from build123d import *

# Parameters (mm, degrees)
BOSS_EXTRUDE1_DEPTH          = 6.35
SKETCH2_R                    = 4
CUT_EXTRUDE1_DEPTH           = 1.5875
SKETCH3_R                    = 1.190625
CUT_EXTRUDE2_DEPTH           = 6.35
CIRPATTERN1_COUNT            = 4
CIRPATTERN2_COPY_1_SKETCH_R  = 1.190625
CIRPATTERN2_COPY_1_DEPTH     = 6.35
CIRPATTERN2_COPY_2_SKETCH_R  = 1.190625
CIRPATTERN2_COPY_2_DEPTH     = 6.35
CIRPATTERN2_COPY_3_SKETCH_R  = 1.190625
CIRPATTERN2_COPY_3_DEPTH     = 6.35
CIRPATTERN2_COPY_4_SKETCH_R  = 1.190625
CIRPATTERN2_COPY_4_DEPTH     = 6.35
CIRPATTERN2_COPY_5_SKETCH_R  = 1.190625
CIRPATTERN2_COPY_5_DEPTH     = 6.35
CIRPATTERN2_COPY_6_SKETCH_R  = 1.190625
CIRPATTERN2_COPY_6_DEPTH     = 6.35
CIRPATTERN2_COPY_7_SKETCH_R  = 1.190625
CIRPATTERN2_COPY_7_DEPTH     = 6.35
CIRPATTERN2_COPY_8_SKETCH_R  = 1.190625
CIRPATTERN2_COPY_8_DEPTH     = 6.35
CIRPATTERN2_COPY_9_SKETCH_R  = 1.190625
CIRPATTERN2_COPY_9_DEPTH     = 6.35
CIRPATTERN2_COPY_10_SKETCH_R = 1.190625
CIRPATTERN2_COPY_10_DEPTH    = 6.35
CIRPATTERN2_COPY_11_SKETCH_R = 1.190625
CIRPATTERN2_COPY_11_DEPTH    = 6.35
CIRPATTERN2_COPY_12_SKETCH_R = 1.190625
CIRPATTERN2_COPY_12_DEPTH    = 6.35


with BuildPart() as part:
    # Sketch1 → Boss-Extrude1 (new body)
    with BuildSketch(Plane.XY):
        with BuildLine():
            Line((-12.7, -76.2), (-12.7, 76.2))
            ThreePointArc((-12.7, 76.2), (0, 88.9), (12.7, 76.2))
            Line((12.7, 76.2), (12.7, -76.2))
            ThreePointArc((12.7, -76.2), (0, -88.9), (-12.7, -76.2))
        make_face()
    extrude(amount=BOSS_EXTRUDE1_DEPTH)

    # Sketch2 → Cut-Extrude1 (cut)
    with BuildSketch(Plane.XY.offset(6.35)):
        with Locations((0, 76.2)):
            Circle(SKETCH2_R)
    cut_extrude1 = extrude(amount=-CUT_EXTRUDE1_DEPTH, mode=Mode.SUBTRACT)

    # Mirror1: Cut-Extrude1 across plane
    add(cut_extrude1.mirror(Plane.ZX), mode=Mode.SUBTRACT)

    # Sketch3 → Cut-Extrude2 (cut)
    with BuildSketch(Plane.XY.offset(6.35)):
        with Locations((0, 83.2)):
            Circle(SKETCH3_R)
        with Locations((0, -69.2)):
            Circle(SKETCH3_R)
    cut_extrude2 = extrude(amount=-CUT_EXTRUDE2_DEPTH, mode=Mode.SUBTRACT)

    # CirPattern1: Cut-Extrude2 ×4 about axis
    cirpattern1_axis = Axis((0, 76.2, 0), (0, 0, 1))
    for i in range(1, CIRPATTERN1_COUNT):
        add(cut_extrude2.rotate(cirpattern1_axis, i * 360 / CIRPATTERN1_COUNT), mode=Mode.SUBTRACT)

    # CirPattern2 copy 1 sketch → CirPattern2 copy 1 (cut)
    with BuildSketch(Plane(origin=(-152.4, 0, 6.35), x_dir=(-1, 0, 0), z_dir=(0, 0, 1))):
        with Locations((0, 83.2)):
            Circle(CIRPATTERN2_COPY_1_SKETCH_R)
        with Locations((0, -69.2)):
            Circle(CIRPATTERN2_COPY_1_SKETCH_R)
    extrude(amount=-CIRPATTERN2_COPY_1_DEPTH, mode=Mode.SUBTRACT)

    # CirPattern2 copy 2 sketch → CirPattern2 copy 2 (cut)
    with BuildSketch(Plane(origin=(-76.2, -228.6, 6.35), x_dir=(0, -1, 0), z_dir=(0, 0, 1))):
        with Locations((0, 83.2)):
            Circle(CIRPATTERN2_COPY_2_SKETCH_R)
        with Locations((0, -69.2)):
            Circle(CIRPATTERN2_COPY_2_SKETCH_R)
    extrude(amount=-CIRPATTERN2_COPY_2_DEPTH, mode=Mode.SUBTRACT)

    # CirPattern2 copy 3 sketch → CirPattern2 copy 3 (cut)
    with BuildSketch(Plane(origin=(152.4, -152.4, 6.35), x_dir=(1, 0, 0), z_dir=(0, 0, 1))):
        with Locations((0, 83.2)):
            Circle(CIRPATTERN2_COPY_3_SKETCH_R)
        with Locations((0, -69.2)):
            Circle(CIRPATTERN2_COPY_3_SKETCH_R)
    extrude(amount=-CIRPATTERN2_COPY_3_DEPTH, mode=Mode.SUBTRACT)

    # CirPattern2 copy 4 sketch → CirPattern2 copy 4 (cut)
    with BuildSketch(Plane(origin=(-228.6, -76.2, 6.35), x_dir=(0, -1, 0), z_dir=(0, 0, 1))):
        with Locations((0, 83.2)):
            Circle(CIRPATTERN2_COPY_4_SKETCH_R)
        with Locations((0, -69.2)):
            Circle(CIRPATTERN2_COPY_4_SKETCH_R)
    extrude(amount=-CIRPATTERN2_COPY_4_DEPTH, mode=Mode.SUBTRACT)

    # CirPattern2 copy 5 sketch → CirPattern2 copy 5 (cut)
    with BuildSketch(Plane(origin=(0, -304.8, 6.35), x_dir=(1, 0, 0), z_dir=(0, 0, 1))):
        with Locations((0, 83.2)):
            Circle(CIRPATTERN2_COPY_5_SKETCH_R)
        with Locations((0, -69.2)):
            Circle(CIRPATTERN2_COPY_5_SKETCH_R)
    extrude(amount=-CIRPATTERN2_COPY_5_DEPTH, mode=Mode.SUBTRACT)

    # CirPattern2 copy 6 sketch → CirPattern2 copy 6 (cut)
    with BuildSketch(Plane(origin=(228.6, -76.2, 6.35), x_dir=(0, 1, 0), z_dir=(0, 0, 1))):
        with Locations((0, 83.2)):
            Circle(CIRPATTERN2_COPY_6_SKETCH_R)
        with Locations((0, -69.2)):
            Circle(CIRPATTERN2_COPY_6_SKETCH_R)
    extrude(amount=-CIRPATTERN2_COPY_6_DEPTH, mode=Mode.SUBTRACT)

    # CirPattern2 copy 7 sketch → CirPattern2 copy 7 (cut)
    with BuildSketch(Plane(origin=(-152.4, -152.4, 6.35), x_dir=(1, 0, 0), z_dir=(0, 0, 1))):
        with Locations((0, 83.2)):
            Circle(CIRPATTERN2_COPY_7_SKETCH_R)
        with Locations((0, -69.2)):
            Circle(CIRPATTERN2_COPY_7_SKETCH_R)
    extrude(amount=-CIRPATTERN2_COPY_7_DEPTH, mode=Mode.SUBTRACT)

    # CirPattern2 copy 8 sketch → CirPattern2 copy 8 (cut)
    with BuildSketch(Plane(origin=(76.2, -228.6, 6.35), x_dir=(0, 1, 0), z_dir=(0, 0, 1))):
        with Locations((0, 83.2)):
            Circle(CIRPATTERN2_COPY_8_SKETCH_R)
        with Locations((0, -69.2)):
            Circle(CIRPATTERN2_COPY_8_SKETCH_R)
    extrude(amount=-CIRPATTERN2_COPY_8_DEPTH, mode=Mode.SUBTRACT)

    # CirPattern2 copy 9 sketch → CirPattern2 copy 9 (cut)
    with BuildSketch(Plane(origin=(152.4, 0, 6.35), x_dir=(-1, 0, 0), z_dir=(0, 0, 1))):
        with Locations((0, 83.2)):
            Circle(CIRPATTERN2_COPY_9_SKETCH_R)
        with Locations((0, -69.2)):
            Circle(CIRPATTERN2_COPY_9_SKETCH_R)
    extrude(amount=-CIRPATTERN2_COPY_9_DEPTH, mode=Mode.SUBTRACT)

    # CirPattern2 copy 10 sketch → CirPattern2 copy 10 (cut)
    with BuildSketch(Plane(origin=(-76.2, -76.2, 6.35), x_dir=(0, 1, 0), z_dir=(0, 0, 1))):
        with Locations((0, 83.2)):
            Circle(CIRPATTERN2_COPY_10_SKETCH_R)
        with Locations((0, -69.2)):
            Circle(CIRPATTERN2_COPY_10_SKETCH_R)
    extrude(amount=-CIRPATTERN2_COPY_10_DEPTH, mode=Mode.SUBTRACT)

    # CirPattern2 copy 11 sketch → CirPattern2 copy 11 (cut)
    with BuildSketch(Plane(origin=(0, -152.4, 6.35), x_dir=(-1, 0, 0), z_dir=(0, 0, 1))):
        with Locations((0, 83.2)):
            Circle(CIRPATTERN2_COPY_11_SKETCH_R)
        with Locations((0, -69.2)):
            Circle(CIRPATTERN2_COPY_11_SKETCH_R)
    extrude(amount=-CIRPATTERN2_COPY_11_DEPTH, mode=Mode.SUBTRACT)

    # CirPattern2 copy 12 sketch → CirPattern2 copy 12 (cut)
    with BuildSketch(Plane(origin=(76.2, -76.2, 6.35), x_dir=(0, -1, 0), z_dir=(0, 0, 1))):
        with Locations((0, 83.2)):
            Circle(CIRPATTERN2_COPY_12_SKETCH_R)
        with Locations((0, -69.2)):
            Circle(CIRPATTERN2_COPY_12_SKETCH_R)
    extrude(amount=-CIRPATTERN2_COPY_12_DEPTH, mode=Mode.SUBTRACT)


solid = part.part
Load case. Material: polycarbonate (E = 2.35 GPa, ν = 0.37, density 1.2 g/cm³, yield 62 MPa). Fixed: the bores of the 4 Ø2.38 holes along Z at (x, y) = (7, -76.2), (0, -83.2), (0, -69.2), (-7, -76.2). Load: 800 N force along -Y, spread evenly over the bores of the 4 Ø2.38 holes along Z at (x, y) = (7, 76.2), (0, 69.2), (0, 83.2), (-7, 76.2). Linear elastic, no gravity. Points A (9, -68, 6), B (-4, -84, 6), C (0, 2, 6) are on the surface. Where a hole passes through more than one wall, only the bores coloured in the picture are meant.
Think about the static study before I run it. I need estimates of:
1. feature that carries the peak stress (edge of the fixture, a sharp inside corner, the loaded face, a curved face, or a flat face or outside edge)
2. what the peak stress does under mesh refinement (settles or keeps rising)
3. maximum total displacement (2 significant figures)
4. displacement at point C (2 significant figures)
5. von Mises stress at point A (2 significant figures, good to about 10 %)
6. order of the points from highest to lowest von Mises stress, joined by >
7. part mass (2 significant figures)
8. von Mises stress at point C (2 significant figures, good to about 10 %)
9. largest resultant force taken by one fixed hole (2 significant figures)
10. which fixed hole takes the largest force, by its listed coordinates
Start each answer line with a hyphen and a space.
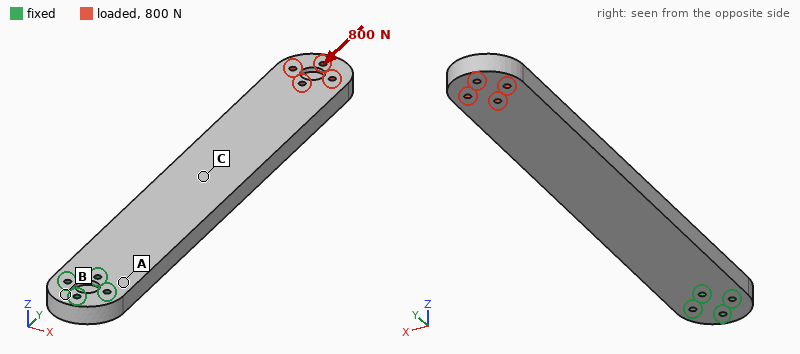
- edge of the fixture
- keeps rising
- 0.34 mm
- 0.16 mm
- 4.1 MPa
- C > A > B
- 33 g
- 5.0 MPa
- 360 N
- (0, -69.2)
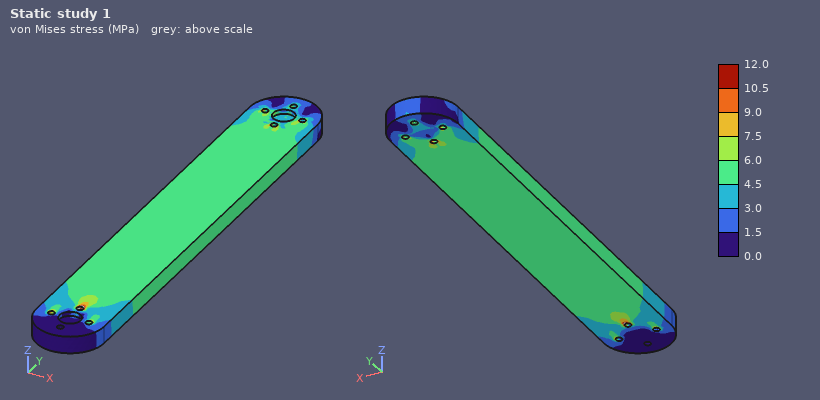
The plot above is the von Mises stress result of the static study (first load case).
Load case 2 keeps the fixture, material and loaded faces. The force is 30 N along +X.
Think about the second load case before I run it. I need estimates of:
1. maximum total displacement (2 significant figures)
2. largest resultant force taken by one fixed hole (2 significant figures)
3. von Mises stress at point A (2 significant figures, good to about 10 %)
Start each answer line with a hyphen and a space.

- 2.0 mm
- 210 N
- 4.6 MPa
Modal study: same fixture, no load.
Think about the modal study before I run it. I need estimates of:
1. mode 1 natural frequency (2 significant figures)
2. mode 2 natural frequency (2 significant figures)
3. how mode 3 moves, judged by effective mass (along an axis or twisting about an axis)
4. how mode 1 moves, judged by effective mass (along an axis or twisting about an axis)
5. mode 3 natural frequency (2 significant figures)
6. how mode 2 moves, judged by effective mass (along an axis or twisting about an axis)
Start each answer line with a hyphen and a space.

- 59 Hz
- 210 Hz
- along Z
- along Z
- 360 Hz
- along X
